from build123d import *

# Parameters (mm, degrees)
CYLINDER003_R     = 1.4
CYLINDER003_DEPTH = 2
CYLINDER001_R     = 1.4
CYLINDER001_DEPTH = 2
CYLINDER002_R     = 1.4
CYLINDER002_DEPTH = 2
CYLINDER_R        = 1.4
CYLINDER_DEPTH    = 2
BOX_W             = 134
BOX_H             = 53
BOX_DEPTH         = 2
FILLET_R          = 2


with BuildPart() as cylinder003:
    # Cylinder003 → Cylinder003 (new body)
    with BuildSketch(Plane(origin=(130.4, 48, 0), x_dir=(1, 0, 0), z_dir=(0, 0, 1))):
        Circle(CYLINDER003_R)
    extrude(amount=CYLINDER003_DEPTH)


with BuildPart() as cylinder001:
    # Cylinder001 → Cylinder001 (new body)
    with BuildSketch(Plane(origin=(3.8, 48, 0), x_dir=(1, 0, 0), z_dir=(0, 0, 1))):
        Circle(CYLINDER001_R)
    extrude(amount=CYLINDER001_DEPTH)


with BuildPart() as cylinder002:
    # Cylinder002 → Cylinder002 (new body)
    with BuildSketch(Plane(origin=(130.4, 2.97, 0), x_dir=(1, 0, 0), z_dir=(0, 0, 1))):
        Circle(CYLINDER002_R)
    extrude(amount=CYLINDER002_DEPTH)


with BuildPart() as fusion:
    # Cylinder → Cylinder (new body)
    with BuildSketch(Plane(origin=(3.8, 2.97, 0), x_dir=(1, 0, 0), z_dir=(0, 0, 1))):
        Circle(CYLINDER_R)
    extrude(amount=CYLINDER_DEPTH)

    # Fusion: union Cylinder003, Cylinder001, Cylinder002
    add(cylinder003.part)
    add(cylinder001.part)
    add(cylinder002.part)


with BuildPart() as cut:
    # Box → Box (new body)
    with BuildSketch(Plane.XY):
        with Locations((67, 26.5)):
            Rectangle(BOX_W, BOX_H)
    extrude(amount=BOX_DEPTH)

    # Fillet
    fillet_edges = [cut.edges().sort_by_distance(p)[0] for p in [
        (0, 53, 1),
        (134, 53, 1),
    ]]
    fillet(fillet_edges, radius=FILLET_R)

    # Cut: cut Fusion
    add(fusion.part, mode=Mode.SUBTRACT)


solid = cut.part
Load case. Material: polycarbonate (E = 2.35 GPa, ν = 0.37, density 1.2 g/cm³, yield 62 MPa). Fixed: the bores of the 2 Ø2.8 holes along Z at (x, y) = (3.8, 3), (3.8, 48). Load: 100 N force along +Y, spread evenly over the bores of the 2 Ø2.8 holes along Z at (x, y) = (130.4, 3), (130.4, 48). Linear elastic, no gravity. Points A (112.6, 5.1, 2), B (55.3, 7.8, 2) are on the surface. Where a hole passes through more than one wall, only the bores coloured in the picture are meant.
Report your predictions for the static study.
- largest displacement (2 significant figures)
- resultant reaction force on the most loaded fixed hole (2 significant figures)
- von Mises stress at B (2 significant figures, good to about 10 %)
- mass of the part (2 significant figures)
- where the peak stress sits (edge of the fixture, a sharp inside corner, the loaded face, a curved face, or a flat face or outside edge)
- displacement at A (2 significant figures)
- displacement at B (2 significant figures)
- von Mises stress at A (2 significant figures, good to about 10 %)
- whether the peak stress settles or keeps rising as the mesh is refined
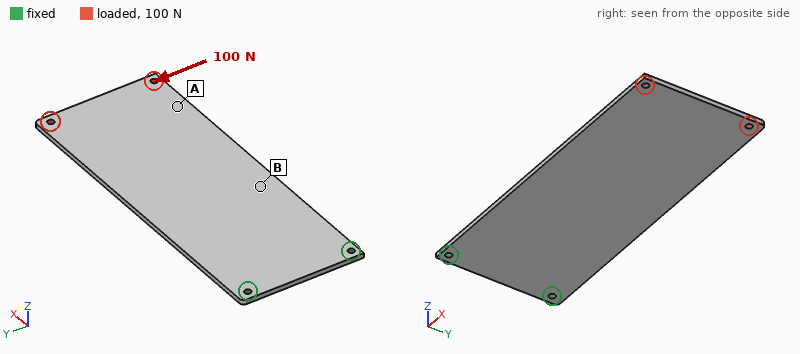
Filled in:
1.5 mm
290 N
5.8 MPa
17 g
edge of the fixture
1.2 mm
0.40 mm
1.7 MPa
keeps rising
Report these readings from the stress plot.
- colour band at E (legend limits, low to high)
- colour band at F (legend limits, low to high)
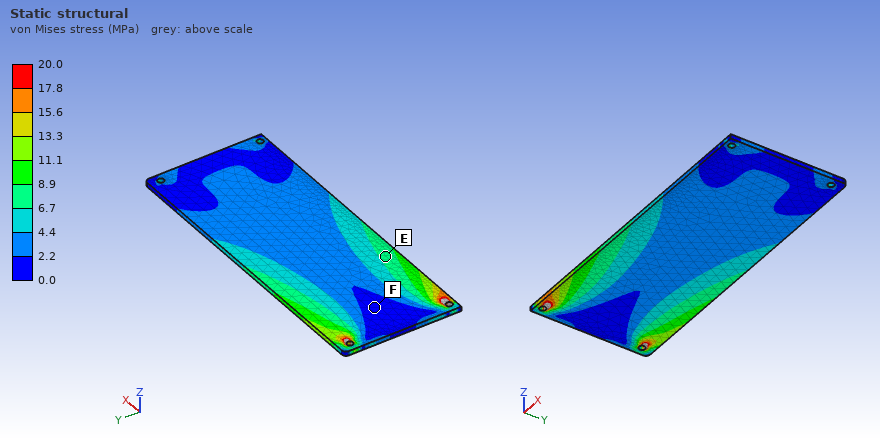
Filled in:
6.7 to 8.9 MPa
0.0 to 2.2 MPa
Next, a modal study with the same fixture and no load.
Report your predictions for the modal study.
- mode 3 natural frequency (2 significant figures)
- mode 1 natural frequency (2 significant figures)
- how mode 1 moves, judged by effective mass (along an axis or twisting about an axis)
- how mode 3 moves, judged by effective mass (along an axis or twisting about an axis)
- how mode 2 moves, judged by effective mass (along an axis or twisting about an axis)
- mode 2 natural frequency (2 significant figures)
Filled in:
160 Hz
25 Hz
along Z
along Z
twisting about X
140 Hz
